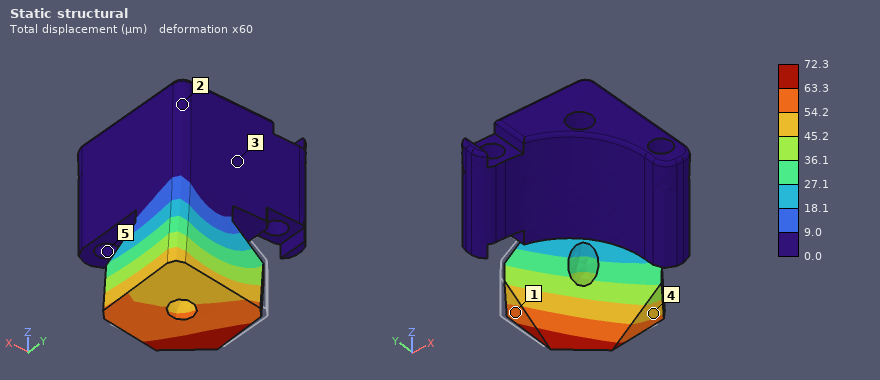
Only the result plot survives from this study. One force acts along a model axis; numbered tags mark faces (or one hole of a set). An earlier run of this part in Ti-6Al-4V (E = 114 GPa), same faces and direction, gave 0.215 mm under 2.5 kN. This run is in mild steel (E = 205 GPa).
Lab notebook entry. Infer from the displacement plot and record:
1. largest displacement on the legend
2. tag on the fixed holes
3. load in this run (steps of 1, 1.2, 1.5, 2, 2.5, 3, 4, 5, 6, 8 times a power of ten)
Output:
72.3 µm
5
1.5 kN
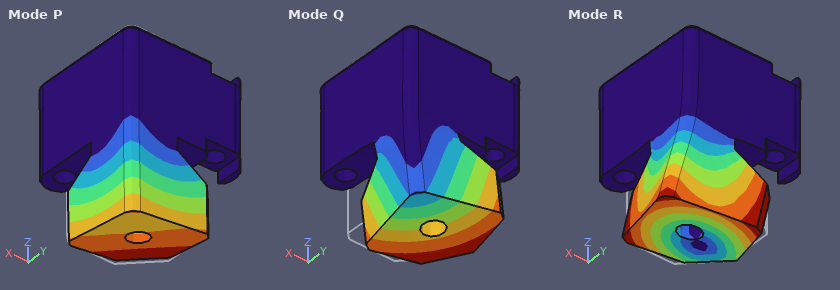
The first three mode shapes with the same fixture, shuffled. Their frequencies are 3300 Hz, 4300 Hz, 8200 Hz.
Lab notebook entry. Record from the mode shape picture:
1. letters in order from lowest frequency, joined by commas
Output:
P, Q, R
